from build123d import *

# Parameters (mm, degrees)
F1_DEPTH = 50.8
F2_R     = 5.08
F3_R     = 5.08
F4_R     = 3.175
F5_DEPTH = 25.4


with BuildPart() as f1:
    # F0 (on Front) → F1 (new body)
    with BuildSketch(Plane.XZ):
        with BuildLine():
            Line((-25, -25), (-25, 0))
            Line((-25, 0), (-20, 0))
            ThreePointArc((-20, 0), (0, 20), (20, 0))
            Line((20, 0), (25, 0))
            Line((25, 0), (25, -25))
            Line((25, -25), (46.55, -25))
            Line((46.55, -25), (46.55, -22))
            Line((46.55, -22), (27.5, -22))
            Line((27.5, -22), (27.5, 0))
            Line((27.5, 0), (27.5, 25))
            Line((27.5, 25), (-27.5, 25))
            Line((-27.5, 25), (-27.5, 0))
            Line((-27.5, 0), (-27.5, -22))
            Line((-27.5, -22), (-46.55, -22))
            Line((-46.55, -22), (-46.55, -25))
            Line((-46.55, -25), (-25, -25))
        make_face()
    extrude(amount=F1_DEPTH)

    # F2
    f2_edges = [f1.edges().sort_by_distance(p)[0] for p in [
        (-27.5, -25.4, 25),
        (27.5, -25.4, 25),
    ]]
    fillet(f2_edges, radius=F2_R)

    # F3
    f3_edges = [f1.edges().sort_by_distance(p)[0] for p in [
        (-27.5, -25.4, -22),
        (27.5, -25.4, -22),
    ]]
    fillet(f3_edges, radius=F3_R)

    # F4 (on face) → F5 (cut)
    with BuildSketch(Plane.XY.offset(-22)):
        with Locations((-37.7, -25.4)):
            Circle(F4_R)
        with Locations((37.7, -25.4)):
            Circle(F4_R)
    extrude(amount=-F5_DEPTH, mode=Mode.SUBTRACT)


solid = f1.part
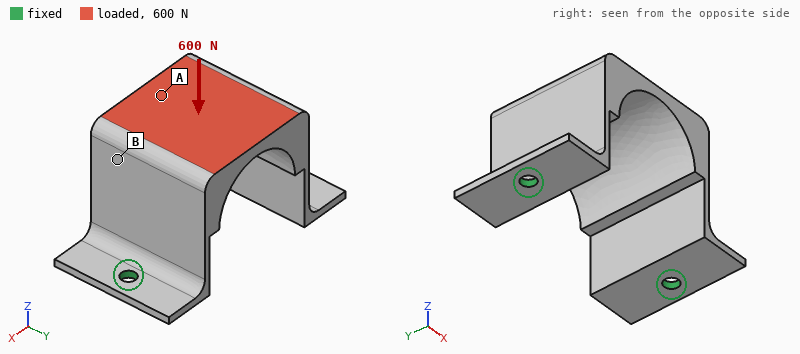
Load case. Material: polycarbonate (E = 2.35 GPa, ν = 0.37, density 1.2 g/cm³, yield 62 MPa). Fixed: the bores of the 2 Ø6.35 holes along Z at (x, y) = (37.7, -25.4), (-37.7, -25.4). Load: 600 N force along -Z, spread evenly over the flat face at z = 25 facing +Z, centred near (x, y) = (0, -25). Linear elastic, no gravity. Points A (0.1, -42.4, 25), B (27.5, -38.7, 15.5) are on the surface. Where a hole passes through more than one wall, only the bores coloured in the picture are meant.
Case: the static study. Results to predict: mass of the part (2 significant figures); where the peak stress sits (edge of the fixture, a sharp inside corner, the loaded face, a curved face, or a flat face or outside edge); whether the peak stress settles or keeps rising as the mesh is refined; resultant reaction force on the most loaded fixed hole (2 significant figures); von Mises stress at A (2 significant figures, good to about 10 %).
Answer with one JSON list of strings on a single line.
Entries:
["60 g", "edge of the fixture", "keeps rising", "320 N", "5.7 MPa"]
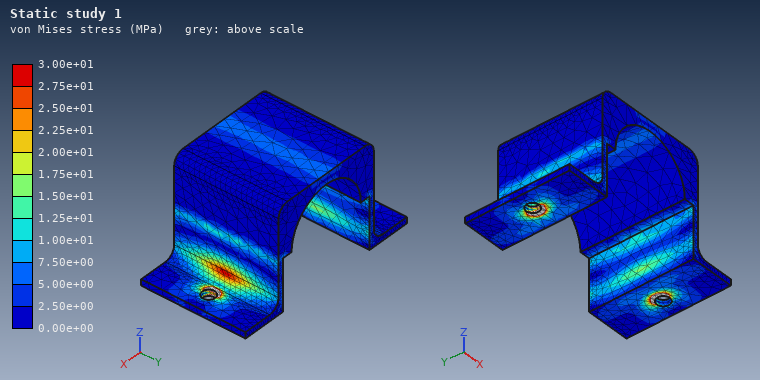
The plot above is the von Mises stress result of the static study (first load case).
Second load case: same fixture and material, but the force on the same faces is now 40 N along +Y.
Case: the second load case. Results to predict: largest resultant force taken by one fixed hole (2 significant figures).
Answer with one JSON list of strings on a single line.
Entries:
["20 N"]
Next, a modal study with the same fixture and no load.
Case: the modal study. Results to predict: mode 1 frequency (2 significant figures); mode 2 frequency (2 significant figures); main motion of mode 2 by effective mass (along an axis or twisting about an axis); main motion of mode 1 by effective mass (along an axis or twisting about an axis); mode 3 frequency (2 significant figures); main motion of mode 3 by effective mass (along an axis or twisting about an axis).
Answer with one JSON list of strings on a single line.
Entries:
["170 Hz", "370 Hz", "along X", "along Y", "630 Hz", "twisting about Z"]
